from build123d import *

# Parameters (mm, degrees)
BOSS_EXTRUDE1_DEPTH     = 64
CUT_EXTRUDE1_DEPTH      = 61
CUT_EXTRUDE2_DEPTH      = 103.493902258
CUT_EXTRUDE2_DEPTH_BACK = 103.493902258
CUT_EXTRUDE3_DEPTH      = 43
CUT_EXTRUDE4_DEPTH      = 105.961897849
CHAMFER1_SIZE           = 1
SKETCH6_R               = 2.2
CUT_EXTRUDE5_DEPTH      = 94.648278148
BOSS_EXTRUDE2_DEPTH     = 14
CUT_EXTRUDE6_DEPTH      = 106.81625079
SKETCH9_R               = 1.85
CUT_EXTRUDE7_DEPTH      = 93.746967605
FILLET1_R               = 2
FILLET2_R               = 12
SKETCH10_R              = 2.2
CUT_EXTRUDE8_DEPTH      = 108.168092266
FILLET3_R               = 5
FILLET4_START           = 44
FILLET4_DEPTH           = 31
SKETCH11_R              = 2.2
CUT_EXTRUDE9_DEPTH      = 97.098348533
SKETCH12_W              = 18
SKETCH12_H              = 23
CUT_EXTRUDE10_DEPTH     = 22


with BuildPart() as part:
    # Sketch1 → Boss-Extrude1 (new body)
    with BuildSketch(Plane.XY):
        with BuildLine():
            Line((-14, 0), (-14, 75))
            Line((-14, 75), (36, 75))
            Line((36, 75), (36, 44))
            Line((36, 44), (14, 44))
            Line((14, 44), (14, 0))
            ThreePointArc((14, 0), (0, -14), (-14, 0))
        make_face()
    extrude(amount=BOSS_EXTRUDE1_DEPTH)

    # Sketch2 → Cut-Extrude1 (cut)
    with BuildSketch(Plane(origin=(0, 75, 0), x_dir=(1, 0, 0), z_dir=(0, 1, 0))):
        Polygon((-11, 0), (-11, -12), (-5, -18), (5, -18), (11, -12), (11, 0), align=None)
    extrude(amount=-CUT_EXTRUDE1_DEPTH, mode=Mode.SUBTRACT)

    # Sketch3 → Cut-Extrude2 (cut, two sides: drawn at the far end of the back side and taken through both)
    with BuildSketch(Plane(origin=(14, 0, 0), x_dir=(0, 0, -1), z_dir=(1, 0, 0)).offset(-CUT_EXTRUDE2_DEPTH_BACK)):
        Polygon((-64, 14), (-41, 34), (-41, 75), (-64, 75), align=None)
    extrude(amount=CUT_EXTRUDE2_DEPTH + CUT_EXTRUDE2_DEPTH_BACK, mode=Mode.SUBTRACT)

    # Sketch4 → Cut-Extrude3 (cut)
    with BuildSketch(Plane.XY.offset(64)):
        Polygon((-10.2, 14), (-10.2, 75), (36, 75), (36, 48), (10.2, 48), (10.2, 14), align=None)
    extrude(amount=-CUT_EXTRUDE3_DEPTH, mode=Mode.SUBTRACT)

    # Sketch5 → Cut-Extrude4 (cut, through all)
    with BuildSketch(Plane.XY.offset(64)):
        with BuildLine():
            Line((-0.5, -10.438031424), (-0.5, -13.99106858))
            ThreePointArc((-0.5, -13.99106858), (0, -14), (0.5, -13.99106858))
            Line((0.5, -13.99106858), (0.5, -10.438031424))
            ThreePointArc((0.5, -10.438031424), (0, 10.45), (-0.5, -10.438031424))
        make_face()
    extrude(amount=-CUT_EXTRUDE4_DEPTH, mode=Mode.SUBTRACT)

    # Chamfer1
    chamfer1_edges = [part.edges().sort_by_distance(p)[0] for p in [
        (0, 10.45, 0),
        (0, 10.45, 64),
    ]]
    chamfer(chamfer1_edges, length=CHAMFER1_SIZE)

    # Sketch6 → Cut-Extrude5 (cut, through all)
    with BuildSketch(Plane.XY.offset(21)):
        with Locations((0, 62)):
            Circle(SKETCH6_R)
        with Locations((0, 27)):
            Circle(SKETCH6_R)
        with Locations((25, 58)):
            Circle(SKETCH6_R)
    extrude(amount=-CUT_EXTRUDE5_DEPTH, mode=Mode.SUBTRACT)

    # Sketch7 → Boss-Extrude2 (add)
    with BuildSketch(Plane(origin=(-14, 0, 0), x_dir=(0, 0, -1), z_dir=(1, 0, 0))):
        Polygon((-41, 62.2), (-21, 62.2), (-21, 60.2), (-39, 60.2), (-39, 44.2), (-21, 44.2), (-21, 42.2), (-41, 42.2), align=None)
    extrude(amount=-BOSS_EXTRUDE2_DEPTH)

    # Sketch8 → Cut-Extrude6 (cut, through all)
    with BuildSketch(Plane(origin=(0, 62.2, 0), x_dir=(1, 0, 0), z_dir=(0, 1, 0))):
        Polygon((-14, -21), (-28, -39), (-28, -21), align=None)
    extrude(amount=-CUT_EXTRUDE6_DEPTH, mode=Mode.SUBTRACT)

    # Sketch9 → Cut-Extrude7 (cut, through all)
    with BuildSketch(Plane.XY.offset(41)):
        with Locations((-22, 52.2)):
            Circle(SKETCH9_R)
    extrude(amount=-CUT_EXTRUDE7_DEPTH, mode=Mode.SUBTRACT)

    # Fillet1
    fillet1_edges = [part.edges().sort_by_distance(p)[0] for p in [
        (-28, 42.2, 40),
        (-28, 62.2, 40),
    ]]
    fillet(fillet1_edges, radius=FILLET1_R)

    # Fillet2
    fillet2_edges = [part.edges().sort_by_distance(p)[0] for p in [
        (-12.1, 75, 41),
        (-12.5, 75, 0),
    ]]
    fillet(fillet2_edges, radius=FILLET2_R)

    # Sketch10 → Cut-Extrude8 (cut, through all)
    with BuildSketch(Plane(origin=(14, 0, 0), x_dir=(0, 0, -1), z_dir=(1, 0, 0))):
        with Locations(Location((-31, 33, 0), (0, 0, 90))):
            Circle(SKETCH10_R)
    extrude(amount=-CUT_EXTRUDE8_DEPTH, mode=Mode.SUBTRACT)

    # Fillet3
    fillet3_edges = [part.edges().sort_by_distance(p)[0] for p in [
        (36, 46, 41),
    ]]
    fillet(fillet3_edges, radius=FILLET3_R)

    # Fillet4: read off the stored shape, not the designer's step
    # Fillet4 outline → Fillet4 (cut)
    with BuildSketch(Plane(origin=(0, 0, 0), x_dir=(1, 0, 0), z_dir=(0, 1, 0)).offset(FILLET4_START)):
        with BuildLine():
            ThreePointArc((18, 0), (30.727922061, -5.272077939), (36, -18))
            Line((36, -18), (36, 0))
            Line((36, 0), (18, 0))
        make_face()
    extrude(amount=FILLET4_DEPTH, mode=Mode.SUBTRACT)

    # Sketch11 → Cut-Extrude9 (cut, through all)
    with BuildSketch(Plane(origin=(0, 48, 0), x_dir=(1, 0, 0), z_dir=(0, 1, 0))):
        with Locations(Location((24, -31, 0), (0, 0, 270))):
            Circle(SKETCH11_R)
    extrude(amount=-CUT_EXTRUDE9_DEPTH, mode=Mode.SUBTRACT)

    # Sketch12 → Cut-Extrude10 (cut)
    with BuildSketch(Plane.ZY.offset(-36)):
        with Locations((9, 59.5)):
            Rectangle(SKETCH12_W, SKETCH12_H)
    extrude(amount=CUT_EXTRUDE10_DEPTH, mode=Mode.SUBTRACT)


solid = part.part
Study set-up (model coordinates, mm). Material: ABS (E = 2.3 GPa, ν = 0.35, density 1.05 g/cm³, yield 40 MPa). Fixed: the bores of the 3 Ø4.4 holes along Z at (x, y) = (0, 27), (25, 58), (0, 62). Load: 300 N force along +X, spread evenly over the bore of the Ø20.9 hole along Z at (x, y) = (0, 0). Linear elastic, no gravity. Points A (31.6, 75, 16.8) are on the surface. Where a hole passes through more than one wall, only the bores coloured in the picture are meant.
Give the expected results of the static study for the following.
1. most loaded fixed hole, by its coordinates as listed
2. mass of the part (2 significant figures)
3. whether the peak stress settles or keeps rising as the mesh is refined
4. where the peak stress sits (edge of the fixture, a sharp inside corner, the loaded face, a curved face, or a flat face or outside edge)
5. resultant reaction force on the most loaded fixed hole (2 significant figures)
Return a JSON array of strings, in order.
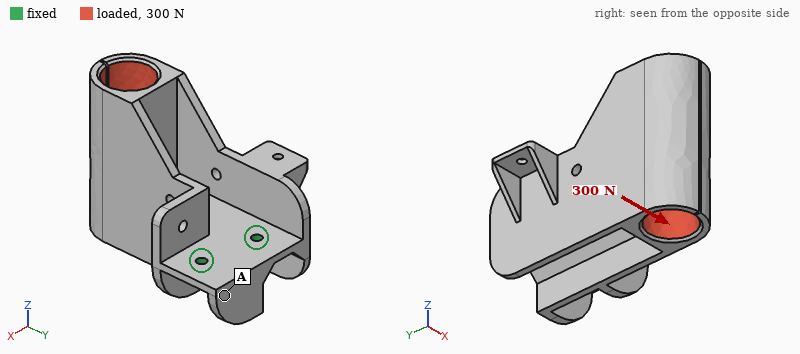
["(0, 27)", "55 g", "keeps rising", "edge of the fixture", "470 N"]
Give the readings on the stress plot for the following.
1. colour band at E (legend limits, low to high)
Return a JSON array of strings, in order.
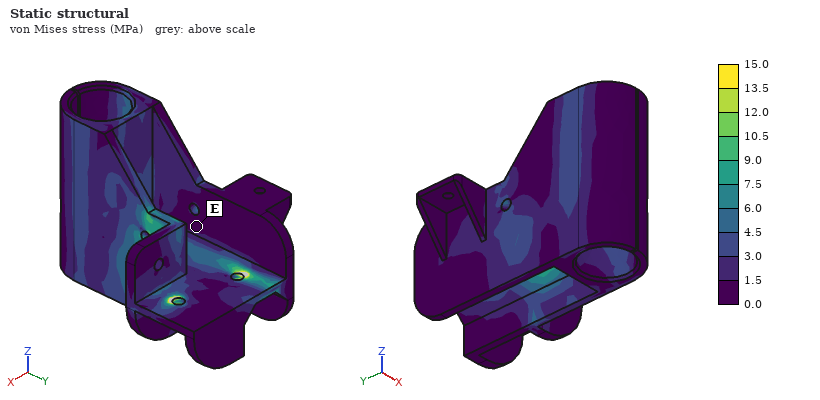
["0.0 to 1.5 MPa"]
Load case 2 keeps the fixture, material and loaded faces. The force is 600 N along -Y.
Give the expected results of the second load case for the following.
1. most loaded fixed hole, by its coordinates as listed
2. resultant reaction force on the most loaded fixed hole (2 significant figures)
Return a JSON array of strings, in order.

["(0, 27)", "460 N"]
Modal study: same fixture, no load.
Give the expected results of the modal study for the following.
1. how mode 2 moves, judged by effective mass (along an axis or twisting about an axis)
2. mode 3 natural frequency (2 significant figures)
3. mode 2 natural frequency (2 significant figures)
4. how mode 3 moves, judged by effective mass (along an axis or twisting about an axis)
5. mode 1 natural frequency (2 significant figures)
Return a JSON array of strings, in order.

["along Z", "1000 Hz", "710 Hz", "along Z", "440 Hz"]
